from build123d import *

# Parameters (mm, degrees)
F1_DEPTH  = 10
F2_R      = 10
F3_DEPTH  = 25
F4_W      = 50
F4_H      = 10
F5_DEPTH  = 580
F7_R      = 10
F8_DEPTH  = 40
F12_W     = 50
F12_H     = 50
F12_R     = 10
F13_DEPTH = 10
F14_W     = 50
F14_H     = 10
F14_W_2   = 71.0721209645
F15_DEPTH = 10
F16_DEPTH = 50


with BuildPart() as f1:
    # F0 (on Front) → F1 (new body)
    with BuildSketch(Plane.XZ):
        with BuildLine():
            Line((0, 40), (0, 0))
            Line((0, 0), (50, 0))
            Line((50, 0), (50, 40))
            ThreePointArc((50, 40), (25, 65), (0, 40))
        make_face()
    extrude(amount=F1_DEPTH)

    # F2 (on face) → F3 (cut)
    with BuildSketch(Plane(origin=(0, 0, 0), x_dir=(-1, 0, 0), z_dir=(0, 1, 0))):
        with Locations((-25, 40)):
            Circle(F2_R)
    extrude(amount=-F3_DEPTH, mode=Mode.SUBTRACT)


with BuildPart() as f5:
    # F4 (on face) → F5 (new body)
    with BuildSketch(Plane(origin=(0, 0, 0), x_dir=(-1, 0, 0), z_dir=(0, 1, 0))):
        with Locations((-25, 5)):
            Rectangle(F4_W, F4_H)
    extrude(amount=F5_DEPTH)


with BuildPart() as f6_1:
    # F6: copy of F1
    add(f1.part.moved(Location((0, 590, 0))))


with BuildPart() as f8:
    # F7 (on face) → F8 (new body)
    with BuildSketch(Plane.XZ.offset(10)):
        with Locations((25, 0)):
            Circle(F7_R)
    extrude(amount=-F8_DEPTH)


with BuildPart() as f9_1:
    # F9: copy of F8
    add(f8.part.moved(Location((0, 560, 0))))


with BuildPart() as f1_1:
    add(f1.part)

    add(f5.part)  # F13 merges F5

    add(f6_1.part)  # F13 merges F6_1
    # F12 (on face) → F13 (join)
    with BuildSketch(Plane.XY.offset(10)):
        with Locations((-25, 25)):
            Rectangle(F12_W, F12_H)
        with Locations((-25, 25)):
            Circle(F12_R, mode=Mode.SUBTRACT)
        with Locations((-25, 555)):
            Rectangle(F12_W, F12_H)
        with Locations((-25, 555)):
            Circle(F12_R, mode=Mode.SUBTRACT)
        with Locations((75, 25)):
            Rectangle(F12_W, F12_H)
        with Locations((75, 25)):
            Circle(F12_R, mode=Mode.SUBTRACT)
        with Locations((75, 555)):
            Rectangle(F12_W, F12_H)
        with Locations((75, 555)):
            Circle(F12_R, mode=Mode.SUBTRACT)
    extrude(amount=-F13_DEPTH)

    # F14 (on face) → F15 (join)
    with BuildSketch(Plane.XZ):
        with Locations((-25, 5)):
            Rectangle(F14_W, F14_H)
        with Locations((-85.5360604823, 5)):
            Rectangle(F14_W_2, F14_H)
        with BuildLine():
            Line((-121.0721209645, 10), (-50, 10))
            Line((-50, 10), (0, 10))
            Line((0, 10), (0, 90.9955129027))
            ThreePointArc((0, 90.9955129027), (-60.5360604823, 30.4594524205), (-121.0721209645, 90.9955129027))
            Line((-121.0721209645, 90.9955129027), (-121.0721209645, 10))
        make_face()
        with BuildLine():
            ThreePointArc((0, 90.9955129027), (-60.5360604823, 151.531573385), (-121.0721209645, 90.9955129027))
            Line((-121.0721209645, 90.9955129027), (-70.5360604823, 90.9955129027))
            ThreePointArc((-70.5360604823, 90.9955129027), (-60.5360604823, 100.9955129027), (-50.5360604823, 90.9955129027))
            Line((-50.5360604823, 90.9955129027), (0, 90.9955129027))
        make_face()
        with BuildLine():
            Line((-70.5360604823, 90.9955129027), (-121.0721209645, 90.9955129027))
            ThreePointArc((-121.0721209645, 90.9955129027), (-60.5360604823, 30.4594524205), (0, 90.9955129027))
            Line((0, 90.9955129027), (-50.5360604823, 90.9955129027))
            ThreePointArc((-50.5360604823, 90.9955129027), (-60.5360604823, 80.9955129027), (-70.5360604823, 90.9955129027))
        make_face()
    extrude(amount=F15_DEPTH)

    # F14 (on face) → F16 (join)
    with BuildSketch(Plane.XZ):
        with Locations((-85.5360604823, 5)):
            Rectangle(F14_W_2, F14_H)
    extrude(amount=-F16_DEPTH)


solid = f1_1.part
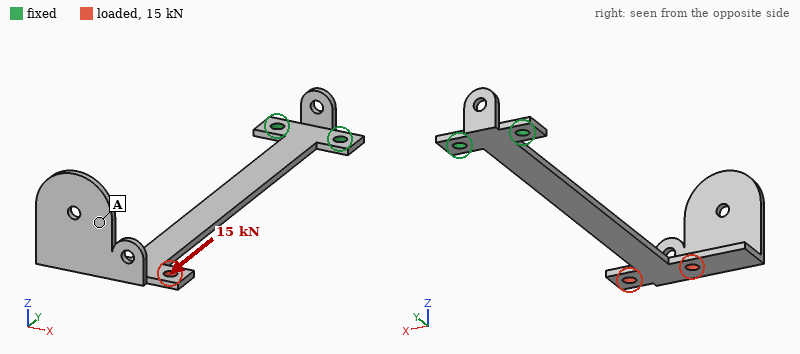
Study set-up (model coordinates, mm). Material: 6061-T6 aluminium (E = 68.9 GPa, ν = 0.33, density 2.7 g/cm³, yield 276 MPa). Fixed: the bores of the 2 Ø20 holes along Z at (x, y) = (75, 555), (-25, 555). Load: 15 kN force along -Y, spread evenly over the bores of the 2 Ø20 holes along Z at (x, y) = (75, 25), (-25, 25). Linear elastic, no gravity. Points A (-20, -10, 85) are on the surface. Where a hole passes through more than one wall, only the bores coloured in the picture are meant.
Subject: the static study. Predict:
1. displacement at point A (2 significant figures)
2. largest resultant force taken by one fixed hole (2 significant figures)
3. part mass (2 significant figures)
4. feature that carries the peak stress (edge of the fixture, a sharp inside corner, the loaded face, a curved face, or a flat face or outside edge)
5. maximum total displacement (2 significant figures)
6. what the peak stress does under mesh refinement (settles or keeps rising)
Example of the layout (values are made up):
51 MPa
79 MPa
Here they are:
0.26 mm
7.7 kN
1.7 kg
a sharp inside corner
0.32 mm
keeps rising
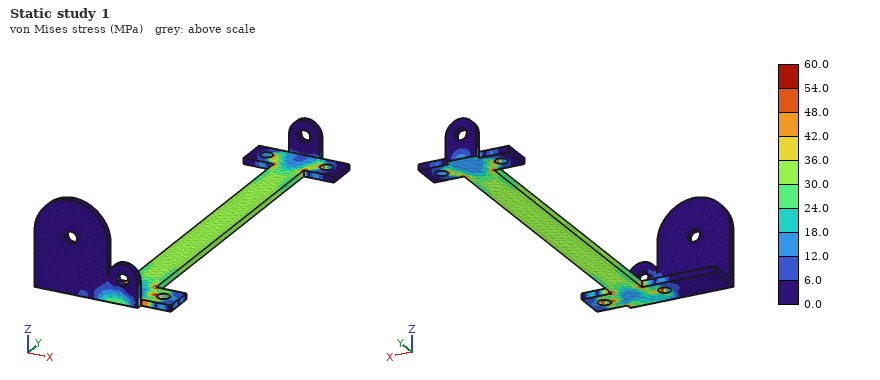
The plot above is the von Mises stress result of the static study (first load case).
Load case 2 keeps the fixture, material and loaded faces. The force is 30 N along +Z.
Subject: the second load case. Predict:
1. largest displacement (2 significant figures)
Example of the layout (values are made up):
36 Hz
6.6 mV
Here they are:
6.0 mm
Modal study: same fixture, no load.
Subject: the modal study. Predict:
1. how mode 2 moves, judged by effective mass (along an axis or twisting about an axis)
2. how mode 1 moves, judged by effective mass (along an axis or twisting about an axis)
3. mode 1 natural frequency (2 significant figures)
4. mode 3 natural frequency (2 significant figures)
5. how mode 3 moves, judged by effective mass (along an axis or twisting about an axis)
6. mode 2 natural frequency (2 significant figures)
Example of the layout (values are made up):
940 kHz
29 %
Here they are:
along X
along Z
12 Hz
77 Hz
along X
49 Hz
